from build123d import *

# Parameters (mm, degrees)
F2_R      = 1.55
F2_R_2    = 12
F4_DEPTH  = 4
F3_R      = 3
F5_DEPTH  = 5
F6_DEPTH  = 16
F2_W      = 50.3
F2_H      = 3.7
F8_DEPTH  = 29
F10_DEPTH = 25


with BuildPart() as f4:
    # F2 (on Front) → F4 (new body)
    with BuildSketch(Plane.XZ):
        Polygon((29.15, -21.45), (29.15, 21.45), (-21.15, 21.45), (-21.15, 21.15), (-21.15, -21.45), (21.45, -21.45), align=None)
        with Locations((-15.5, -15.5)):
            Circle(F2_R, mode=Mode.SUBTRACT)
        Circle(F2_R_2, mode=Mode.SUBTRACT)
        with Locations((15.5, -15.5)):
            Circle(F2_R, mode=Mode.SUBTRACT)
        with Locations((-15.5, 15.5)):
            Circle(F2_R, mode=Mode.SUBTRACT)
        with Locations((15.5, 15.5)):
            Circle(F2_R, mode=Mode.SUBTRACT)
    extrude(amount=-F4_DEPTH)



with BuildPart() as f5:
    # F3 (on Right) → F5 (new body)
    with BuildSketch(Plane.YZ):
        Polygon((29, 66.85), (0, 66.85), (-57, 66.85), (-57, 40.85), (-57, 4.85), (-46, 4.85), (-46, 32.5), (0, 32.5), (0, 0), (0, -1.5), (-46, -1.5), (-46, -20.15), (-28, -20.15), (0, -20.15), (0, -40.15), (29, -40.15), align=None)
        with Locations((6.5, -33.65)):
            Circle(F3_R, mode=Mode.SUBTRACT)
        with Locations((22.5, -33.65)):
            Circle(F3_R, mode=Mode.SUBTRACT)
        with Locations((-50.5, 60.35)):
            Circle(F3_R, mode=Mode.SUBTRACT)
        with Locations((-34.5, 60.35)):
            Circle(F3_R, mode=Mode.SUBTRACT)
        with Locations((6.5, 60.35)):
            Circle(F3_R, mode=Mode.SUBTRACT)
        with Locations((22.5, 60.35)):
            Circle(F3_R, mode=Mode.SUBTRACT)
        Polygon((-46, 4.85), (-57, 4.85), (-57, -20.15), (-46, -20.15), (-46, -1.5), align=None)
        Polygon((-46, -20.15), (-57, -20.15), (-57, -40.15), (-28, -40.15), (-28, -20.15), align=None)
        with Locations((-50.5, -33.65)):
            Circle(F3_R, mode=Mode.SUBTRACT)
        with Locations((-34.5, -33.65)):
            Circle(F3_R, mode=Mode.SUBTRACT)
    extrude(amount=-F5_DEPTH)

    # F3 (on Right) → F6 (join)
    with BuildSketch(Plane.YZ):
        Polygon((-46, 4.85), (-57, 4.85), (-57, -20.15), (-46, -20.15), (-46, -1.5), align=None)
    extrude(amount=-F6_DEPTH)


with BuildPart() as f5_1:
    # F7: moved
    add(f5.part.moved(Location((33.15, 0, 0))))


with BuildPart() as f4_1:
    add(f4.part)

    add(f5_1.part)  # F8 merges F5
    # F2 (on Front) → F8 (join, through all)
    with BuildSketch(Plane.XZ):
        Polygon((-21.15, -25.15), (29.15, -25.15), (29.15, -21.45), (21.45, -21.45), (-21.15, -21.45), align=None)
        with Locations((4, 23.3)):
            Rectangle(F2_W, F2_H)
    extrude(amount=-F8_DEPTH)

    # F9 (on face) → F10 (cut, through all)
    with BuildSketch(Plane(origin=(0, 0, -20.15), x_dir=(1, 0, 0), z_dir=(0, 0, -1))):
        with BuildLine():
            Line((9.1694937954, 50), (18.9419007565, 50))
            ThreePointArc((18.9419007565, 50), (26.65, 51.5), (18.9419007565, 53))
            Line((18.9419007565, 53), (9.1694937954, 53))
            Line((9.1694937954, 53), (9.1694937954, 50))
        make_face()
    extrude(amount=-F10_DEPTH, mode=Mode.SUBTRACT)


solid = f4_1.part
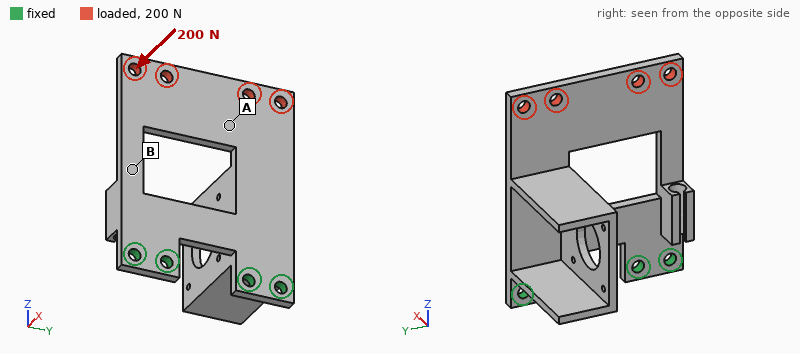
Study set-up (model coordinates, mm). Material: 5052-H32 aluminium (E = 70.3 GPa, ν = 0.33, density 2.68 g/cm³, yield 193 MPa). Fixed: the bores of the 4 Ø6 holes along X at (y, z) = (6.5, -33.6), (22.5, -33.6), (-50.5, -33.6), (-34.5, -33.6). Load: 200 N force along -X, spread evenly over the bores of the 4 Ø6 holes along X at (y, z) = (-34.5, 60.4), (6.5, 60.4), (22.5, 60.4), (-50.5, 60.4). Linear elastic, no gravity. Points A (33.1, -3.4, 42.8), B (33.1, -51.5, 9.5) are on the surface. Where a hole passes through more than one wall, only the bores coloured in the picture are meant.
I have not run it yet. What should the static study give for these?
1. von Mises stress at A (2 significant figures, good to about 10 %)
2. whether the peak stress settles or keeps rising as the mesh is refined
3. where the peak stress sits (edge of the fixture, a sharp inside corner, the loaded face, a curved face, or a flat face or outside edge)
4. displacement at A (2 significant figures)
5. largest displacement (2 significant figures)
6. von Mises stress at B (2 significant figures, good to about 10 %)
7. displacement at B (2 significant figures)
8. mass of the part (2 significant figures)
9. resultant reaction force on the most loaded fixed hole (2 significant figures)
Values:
13 MPa
keeps rising
edge of the fixture
0.49 mm
0.86 mm
52 MPa
0.17 mm
140 g
180 N
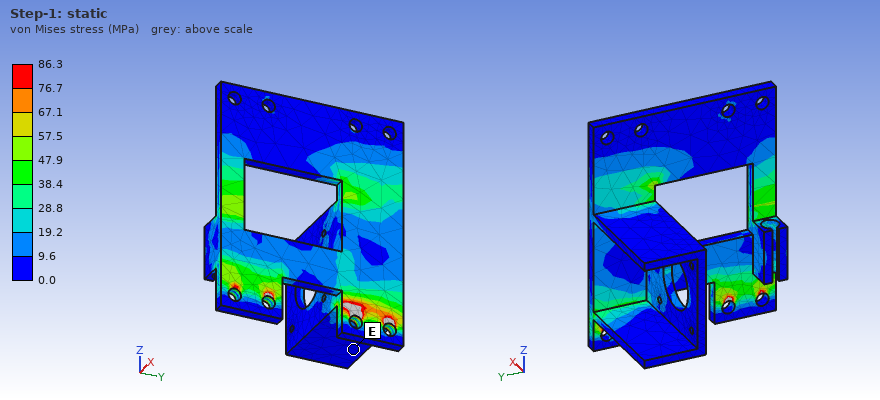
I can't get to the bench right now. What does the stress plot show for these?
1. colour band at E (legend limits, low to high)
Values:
0.0 to 9.6 MPa
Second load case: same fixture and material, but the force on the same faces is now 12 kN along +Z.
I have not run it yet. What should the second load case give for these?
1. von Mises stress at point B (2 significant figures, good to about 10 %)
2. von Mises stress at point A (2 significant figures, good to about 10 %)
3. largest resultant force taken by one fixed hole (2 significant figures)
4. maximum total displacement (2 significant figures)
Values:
89 MPa
30 MPa
4.0 kN
0.20 mm
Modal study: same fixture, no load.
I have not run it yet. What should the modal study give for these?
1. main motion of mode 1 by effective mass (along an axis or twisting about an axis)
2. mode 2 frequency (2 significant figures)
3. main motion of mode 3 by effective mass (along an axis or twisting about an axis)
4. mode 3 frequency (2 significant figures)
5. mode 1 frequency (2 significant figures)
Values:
along X
980 Hz
along Y
1700 Hz
430 Hz
